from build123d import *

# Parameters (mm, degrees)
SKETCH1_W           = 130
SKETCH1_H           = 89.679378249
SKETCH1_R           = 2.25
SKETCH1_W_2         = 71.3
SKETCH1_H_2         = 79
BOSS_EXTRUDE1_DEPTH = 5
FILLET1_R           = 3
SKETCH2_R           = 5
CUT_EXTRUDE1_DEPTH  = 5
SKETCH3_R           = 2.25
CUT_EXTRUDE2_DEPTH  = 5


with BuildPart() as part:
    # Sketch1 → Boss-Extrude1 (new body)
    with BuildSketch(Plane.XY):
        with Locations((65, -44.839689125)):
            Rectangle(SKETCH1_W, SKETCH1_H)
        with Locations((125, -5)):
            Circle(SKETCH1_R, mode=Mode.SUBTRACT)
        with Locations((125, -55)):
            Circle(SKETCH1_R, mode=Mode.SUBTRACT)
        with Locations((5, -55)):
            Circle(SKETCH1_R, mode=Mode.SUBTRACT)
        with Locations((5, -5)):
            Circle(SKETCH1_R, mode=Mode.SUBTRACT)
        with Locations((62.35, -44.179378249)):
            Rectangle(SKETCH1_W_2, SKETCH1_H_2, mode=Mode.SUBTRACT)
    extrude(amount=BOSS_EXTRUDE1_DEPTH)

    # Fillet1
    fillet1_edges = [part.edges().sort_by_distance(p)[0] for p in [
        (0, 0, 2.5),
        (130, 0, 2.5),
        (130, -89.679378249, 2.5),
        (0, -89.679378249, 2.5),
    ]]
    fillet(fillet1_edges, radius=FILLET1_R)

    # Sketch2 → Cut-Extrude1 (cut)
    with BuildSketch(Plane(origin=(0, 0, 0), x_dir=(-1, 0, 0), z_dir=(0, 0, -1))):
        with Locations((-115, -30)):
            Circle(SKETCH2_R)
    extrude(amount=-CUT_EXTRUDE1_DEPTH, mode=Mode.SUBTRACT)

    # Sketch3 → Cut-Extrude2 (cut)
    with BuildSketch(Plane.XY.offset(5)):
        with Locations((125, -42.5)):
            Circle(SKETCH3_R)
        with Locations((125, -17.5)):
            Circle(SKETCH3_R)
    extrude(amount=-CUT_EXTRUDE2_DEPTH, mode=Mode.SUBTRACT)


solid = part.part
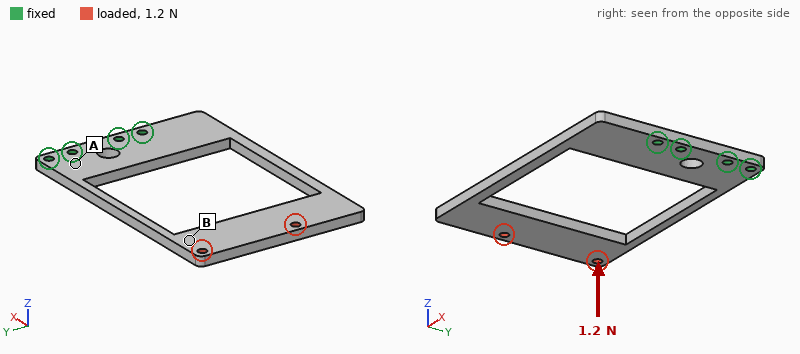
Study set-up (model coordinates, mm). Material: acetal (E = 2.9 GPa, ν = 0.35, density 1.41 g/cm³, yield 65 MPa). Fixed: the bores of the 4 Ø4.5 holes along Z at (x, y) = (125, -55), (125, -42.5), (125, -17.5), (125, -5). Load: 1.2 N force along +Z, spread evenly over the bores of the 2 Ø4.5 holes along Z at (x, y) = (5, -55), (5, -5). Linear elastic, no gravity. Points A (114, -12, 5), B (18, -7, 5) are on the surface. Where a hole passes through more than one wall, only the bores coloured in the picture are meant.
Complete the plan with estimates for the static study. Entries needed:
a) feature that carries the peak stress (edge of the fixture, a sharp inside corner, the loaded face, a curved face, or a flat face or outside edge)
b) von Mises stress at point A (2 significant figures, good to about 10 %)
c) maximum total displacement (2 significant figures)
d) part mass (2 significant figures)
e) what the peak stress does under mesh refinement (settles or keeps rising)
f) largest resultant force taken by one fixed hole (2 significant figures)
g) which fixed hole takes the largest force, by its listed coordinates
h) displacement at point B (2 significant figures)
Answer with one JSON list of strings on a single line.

["a sharp inside corner", "0.54 MPa", "1.6 mm", "41 g", "keeps rising", "0.53 N", "(125, -55)", "1.2 mm"]
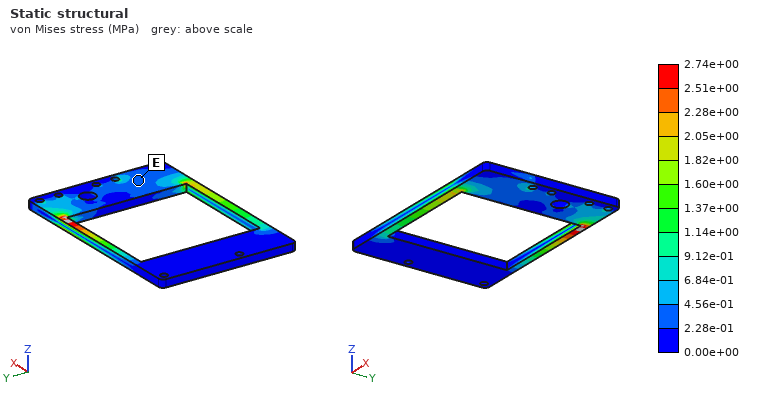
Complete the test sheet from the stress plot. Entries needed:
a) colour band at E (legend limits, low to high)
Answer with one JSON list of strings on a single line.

["2.28e-01 to 4.56e-01 MPa"]
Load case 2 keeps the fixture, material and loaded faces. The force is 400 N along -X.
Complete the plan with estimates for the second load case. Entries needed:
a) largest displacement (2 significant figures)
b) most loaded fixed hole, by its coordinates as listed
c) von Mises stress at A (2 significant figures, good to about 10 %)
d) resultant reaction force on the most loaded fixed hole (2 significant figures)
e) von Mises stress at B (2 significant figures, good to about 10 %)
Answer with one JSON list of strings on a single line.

["0.45 mm", "(125, -55)", "2.5 MPa", "240 N", "4.4 MPa"]
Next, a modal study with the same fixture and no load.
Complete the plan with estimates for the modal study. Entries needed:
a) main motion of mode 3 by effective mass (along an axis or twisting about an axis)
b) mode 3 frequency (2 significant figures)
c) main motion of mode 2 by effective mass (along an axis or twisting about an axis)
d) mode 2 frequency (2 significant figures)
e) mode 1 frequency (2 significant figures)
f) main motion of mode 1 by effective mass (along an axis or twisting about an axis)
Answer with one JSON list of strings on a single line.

["twisting about X", "130 Hz", "along Y", "110 Hz", "40 Hz", "along Z"]
